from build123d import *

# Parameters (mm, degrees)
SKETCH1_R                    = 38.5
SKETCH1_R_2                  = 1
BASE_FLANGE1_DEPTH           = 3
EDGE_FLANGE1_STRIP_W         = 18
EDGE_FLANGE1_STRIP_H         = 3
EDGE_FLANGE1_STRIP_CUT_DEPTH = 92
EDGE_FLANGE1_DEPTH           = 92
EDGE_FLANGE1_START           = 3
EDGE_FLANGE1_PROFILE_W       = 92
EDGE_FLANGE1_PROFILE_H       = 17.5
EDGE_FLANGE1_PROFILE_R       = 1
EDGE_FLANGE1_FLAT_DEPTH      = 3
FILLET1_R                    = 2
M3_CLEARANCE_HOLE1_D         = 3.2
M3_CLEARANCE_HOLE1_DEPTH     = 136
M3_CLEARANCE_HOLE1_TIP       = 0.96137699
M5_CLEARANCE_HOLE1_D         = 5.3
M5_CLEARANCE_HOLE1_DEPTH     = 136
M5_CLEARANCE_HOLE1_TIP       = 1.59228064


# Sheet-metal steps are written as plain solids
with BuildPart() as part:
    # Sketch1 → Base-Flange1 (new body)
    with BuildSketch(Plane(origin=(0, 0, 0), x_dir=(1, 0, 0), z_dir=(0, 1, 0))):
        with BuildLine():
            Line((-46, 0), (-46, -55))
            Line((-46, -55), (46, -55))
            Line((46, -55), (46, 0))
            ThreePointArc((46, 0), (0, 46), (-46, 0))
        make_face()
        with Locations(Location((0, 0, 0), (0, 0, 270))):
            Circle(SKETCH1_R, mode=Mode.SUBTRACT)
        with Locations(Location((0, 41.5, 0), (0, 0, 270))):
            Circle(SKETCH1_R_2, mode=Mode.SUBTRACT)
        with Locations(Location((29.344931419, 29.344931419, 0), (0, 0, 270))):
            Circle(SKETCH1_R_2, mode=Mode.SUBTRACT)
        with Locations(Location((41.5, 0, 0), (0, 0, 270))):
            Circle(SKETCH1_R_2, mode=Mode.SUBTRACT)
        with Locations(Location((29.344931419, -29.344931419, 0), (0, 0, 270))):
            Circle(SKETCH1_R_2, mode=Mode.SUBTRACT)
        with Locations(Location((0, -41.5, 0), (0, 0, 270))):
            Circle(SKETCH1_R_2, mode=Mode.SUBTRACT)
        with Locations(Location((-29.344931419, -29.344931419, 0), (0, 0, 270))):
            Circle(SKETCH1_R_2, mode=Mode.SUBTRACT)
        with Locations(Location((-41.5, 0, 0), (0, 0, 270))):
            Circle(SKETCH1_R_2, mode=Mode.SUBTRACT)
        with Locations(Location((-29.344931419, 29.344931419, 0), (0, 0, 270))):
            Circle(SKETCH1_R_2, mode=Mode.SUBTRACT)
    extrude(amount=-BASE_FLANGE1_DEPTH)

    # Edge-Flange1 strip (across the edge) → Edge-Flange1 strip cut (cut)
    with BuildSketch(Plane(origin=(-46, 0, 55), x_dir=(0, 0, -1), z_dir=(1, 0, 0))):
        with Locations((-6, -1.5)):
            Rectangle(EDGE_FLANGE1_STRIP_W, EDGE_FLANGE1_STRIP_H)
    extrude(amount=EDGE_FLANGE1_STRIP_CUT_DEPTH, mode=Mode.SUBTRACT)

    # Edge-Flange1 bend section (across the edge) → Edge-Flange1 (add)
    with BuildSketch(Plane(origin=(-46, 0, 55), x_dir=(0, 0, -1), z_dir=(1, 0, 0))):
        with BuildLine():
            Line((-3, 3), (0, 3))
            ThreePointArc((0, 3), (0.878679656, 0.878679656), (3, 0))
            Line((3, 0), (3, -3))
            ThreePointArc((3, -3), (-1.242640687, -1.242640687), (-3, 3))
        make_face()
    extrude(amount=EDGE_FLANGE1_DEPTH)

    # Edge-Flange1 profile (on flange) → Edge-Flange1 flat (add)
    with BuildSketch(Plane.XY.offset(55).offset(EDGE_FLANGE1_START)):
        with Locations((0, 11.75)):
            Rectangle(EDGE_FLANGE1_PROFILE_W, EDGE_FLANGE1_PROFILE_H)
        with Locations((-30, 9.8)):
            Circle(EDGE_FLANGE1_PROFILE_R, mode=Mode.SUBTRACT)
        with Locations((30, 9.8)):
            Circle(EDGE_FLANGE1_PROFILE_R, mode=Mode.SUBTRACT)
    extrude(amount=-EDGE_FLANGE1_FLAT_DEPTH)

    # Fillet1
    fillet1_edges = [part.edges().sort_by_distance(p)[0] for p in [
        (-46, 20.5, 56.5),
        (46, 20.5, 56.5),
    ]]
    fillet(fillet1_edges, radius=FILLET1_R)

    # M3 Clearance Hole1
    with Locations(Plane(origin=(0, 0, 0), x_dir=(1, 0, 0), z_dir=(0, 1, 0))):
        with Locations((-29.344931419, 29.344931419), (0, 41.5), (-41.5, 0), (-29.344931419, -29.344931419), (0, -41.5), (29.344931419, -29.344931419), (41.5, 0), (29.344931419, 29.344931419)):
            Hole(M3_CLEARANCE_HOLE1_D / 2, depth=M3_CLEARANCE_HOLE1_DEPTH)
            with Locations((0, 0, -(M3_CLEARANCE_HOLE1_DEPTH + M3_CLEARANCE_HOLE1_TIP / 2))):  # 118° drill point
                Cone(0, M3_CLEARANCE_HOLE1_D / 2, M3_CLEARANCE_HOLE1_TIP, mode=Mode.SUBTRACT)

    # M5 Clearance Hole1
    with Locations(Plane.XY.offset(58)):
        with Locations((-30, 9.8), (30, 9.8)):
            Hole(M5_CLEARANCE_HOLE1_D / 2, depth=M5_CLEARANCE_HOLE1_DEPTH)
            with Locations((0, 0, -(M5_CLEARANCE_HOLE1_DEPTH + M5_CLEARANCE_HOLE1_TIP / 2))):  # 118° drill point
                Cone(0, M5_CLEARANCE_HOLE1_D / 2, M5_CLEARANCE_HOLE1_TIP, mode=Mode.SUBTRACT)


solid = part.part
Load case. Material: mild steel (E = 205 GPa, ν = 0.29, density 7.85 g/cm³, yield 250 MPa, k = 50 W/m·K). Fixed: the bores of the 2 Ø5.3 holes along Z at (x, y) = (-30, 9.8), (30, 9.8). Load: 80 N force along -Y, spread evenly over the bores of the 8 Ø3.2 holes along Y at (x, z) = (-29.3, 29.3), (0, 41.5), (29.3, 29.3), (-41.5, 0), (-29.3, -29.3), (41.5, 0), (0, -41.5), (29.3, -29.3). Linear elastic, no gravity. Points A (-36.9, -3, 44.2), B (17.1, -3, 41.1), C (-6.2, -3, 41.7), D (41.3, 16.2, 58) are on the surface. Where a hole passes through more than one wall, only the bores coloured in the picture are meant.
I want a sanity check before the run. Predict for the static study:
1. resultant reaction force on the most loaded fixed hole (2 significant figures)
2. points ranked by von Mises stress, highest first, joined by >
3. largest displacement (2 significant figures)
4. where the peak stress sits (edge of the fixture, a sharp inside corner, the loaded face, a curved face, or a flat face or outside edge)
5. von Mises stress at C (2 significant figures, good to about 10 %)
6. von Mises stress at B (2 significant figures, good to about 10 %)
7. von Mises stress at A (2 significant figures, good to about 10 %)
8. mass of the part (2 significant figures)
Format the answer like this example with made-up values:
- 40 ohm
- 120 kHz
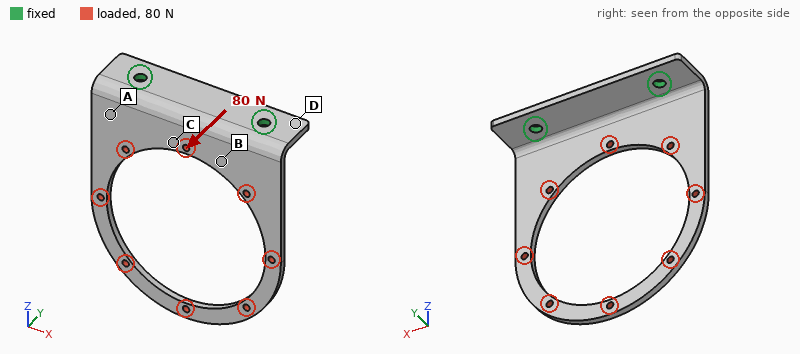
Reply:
- 40 N
- A > B > C > D
- 0.88 mm
- the loaded face
- 14 MPa
- 25 MPa
- 34 MPa
- 130 g
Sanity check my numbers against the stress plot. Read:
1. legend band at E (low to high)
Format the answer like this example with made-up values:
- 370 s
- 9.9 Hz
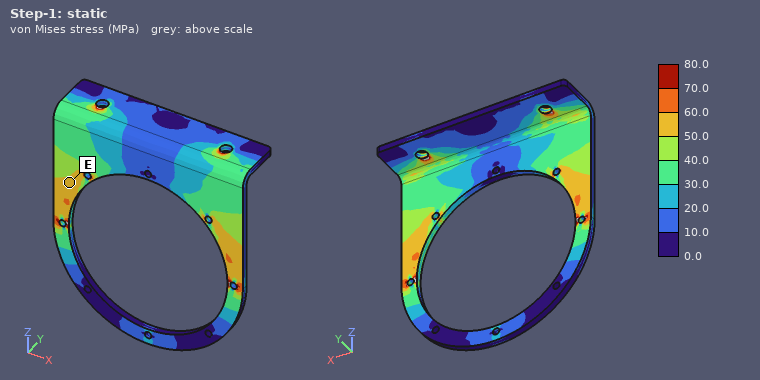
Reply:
- 50.0 to 60.0 MPa
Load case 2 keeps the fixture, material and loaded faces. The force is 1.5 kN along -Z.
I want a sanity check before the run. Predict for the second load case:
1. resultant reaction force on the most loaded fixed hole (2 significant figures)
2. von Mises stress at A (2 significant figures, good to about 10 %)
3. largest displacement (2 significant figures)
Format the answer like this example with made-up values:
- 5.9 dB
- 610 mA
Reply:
- 790 N
- 22 MPa
- 0.31 mm
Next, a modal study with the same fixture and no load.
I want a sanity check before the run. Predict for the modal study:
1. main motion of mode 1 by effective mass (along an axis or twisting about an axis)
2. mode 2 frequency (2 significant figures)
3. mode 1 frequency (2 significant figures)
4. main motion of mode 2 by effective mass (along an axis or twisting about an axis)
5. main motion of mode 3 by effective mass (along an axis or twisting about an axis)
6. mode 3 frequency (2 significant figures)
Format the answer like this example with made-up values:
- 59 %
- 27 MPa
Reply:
- along Y
- 650 Hz
- 270 Hz
- twisting about Z
- along Y
- 1200 Hz
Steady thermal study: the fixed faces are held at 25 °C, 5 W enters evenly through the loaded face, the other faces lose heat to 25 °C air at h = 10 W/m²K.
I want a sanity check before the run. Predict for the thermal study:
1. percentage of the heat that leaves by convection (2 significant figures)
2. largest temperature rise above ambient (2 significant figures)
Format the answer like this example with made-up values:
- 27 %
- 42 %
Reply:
- 38 %
- 51 K
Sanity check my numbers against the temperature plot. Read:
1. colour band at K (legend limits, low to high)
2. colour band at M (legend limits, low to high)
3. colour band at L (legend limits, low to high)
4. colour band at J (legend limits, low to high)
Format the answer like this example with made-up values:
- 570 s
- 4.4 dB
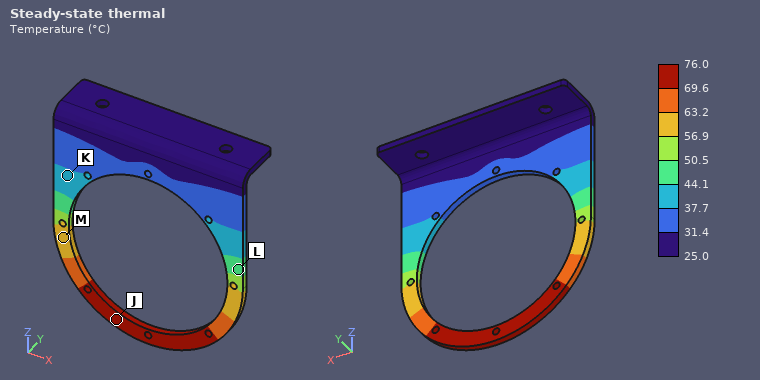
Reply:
- 37.7 to 44.1 °C
- 56.9 to 63.2 °C
- 44.1 to 50.5 °C
- 69.6 to 76.0 °C
